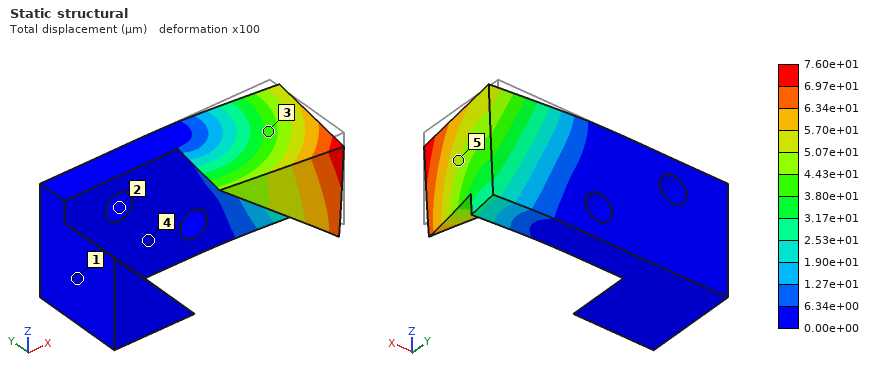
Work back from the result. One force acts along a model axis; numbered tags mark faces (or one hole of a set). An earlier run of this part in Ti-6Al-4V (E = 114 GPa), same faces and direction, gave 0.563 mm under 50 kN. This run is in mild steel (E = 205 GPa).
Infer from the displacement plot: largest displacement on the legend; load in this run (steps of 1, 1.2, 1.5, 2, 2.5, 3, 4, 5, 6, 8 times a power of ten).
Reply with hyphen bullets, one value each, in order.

- 7.60e+01 µm
- 12 kN
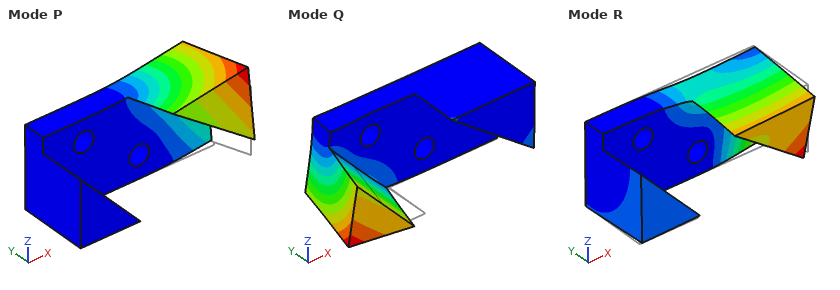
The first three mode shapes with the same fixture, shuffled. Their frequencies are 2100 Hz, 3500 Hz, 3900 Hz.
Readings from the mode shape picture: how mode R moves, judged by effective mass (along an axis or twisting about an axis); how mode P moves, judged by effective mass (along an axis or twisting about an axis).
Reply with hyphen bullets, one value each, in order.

- along Z
- along Y
